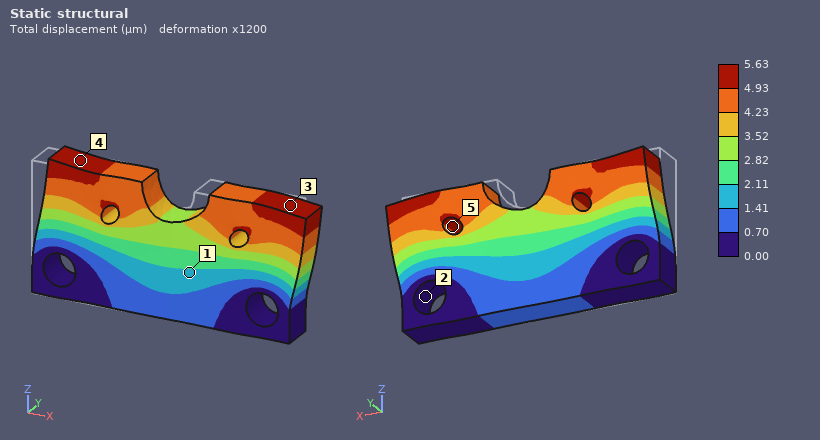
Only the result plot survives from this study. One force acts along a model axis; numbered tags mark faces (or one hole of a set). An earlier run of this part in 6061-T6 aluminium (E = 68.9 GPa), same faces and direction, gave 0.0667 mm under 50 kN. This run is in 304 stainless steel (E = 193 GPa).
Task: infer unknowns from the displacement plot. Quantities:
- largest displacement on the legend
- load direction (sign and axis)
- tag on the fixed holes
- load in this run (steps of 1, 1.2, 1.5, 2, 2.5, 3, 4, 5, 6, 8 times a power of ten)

5.63 µm
+X
2
12 kN
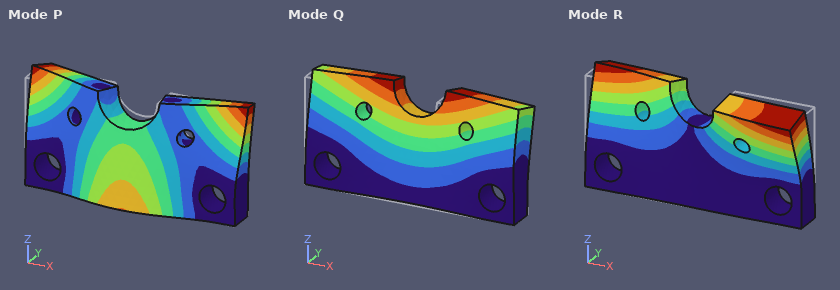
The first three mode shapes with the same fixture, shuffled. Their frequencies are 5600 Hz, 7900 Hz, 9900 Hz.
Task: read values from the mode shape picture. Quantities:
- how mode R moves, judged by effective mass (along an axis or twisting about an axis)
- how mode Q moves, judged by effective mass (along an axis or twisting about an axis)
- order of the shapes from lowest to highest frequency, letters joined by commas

twisting about Z
along Y
Q, R, P
